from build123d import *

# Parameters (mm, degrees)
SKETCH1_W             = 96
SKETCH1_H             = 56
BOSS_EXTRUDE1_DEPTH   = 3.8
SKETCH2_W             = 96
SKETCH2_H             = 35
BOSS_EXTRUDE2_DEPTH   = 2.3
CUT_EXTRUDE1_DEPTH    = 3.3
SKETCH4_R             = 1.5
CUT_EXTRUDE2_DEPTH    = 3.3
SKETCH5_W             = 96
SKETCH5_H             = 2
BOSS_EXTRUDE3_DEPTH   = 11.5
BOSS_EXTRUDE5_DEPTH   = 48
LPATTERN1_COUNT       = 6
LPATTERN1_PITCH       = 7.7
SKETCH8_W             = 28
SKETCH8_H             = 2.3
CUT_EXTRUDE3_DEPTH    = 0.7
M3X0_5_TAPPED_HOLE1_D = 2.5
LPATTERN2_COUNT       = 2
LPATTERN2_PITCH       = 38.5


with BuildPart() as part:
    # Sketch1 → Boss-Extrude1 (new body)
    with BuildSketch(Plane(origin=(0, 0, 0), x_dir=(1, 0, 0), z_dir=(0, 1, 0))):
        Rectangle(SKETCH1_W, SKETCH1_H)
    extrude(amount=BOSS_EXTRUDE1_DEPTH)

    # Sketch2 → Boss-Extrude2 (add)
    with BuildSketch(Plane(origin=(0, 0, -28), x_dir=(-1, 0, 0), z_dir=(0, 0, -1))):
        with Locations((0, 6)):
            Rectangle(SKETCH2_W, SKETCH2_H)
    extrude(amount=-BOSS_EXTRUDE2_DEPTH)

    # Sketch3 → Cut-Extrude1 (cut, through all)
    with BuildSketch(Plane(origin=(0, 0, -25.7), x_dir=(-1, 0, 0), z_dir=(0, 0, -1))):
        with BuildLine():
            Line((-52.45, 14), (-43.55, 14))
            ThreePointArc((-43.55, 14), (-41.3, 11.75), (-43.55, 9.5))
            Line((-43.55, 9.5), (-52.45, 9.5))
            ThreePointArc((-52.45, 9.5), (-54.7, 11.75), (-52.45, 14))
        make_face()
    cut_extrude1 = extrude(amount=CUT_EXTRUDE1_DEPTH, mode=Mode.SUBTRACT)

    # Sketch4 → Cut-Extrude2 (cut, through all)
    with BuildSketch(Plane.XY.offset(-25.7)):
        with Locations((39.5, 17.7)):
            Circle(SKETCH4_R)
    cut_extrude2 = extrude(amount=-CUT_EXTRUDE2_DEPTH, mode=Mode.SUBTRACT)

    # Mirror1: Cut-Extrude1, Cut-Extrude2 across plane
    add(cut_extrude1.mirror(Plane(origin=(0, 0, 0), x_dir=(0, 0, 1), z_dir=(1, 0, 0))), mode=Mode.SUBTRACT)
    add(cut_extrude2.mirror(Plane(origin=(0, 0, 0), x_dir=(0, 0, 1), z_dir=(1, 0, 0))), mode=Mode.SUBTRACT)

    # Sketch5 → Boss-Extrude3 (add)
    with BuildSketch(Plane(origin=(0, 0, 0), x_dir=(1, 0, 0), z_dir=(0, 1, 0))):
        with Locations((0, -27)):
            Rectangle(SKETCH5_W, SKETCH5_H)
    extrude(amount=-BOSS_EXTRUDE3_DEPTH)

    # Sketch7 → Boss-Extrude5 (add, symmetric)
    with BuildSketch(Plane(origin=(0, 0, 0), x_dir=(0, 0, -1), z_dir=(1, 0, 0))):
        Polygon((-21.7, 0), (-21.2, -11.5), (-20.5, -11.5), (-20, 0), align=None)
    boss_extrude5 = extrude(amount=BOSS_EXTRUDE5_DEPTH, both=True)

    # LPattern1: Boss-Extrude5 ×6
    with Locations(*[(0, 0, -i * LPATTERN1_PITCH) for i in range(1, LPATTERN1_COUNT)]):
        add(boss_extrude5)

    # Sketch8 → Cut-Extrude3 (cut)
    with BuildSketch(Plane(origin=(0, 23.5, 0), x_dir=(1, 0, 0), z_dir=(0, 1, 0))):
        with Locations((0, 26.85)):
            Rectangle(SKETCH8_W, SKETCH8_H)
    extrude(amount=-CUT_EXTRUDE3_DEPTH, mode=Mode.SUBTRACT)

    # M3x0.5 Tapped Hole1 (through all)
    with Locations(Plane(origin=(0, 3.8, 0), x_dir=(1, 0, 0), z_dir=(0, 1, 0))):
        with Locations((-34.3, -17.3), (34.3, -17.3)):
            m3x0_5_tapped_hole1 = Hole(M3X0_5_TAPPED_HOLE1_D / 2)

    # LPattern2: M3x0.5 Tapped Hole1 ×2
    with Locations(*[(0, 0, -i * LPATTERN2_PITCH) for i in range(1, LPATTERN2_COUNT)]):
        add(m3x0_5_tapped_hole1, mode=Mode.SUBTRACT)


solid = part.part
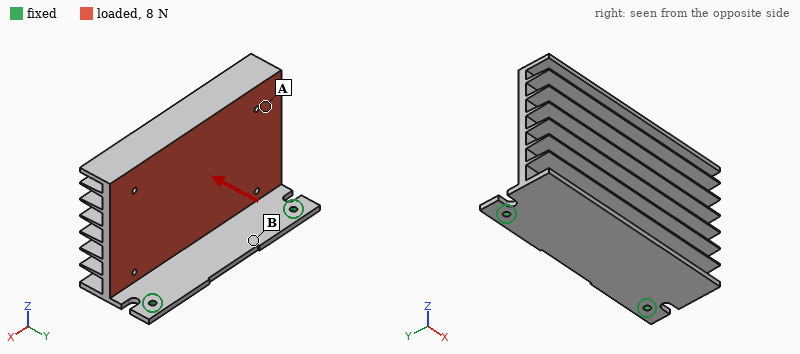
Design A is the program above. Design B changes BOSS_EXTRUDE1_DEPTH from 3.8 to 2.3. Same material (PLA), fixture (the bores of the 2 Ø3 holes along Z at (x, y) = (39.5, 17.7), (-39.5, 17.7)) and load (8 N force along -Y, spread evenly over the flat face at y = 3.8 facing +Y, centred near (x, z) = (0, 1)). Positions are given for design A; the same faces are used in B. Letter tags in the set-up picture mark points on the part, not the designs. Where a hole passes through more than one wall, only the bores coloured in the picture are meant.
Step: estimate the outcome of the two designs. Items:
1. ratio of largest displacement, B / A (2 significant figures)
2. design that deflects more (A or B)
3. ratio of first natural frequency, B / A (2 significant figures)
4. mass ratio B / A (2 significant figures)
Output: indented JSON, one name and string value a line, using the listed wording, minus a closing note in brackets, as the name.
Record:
{
  "ratio of largest displacement, B / A": "1.3",
  "design that deflects more": "B",
  "ratio of first natural frequency, B / A": "1.0",
  "mass ratio B / A": "0.79"
}
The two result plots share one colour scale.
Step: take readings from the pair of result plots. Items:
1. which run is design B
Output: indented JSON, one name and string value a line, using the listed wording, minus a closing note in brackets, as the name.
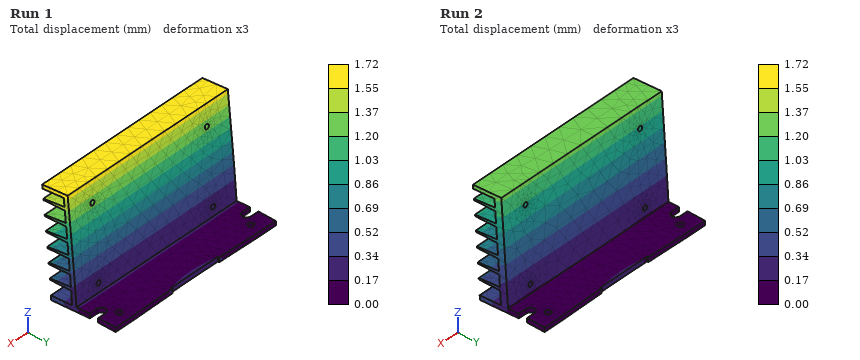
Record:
{
  "which run is design B": "Run 1"
}
